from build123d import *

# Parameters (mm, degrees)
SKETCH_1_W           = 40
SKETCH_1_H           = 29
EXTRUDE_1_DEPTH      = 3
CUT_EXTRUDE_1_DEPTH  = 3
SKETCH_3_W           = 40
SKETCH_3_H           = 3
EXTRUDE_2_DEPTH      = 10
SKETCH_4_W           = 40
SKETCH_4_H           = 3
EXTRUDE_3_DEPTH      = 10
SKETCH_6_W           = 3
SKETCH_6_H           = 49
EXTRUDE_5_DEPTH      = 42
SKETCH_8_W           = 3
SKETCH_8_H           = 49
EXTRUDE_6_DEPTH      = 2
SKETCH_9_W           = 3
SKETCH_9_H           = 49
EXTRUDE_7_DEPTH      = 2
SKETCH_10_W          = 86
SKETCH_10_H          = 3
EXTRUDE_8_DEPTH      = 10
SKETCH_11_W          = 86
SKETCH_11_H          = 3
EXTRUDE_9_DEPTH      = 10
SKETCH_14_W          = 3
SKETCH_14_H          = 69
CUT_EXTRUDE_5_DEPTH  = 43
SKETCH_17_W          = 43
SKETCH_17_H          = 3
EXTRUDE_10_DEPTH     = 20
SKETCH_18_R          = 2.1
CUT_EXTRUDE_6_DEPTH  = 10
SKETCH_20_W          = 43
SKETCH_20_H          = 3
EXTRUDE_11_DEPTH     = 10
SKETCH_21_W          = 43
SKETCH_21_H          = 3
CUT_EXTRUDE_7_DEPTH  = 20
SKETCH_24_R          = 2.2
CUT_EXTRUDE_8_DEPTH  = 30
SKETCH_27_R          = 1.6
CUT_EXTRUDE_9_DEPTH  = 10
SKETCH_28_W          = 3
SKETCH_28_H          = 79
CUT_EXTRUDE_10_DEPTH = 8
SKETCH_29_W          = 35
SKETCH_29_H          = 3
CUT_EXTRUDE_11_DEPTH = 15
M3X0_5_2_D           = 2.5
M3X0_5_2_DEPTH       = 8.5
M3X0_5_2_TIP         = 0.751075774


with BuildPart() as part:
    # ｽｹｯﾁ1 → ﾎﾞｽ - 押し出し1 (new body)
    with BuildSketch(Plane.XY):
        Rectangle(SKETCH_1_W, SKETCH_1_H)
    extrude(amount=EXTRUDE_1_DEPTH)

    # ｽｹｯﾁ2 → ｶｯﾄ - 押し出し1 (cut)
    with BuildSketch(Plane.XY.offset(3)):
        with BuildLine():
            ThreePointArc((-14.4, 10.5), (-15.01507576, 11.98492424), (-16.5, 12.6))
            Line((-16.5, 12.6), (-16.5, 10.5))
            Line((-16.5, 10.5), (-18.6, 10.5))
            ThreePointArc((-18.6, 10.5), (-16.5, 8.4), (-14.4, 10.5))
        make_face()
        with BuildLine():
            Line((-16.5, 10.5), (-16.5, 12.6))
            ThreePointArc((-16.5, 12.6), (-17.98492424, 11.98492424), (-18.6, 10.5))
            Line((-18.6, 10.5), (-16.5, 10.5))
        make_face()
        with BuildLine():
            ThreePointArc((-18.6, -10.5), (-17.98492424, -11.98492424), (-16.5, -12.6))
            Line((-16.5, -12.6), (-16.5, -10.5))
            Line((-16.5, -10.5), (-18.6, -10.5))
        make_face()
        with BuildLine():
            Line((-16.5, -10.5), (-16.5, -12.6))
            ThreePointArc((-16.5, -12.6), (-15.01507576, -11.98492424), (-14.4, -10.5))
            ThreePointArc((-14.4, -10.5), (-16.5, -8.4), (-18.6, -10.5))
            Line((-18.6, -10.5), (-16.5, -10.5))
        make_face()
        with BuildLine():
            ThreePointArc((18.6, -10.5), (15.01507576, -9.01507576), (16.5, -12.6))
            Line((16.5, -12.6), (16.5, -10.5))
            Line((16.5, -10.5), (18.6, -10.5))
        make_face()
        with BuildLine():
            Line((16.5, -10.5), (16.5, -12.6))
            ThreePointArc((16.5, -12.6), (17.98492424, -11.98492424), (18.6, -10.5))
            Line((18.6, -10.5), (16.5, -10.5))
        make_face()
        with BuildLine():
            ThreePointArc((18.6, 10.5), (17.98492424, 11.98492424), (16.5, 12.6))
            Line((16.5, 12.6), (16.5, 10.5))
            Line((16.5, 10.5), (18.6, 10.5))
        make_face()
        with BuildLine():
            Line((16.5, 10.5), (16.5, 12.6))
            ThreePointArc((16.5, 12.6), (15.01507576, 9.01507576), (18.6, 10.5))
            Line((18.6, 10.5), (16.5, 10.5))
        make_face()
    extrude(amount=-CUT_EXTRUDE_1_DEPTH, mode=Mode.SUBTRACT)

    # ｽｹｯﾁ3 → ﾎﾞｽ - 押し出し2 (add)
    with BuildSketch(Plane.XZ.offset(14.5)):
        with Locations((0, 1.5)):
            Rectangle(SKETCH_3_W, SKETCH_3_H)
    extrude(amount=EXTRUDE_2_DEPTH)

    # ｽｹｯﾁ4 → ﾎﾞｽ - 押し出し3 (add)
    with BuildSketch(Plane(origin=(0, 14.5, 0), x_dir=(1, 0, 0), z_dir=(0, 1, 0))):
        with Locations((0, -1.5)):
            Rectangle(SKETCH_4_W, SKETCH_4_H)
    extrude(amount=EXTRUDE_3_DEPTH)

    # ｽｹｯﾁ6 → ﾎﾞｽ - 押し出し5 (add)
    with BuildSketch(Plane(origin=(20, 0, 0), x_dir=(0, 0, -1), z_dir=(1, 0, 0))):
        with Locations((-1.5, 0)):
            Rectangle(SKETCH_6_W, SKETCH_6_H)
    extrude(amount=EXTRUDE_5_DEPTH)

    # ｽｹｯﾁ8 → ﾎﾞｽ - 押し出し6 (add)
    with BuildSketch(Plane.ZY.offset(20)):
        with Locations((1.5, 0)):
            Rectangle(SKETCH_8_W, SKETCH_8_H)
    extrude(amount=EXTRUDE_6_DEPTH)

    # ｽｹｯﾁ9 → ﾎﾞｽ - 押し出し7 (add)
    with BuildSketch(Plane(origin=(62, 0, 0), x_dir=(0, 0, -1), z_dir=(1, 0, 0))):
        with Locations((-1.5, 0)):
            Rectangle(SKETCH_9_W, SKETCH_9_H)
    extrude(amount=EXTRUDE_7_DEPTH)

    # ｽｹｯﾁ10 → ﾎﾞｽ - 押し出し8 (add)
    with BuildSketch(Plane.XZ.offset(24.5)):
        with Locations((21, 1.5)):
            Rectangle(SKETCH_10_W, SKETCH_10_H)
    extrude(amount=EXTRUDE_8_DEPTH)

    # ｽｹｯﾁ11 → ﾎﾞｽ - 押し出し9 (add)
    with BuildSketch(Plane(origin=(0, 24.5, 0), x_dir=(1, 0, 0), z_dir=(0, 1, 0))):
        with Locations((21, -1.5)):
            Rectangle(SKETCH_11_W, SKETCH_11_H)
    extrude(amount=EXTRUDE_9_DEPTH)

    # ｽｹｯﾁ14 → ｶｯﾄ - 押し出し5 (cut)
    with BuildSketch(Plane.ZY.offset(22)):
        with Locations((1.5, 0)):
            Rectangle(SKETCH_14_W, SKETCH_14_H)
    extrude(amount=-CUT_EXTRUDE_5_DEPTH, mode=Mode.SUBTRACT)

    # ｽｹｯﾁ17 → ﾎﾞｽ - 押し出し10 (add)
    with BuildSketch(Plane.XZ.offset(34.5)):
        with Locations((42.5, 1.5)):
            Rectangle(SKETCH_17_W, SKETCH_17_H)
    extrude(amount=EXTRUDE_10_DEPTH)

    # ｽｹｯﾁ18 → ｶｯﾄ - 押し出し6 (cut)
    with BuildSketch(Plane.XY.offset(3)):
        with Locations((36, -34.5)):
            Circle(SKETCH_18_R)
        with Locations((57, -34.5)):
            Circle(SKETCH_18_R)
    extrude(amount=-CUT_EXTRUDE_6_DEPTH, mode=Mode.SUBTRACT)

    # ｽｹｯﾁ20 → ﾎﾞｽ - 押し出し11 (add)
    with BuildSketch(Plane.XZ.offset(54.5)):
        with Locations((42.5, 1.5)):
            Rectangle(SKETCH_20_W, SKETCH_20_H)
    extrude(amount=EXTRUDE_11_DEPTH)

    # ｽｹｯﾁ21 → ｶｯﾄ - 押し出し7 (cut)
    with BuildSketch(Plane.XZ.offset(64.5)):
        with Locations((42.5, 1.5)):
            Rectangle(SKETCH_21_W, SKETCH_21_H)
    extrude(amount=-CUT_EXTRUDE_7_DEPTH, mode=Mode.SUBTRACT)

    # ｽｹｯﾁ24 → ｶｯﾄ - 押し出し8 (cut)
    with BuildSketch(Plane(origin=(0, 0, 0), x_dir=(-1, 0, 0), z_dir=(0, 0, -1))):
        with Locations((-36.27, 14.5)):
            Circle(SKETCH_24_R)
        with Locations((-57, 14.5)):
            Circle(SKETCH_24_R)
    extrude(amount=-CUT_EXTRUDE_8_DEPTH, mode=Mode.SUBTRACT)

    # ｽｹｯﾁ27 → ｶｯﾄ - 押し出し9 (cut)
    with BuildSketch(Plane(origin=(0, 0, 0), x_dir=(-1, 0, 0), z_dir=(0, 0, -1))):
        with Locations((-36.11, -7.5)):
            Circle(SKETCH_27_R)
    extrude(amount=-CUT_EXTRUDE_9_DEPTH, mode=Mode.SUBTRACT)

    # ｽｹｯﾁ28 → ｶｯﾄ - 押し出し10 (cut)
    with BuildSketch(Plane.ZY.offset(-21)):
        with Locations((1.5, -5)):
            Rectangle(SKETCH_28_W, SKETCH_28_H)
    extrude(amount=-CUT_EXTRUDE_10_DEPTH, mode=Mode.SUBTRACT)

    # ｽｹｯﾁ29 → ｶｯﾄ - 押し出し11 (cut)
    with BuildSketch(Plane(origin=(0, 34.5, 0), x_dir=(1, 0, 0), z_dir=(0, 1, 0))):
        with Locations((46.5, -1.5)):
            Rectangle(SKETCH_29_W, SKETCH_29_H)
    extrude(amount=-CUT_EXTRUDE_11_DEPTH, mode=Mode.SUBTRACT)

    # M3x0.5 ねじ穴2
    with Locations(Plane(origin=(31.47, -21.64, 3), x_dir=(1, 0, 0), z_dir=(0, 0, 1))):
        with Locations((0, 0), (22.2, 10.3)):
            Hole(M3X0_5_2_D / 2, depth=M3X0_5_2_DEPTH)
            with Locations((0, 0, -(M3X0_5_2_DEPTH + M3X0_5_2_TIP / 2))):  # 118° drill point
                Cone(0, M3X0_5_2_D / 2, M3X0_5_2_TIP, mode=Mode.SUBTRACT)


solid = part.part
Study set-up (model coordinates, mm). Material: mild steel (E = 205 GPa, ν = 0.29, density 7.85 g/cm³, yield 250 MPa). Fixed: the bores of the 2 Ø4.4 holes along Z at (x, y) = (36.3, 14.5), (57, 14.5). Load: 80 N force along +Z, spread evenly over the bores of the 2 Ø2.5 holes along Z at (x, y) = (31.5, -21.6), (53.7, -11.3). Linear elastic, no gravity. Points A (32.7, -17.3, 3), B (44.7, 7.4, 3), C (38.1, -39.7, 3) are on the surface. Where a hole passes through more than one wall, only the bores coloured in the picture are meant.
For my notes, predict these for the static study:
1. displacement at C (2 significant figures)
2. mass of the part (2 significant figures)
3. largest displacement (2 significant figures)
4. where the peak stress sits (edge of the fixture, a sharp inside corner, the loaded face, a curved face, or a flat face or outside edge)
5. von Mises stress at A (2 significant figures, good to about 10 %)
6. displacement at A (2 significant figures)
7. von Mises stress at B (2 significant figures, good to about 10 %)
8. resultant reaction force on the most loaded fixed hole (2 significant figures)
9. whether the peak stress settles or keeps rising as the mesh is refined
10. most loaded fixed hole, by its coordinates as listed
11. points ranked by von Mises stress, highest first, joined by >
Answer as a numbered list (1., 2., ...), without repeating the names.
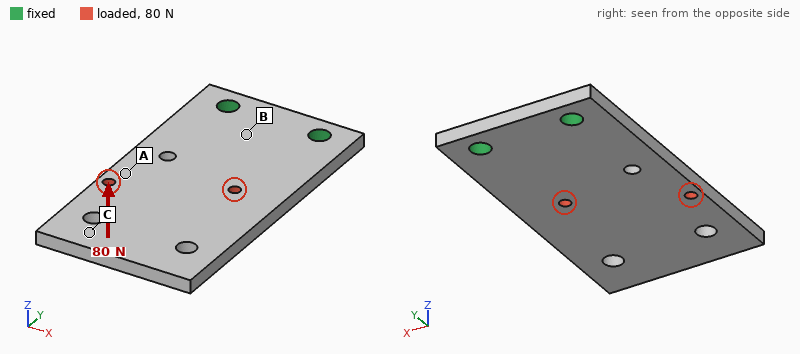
1. 0.10 mm
2. 51 g
3. 0.12 mm
4. edge of the fixture
5. 11 MPa
6. 0.053 mm
7. 31 MPa
8. 53 N
9. keeps rising
10. (36.3, 14.5)
11. B > A > C
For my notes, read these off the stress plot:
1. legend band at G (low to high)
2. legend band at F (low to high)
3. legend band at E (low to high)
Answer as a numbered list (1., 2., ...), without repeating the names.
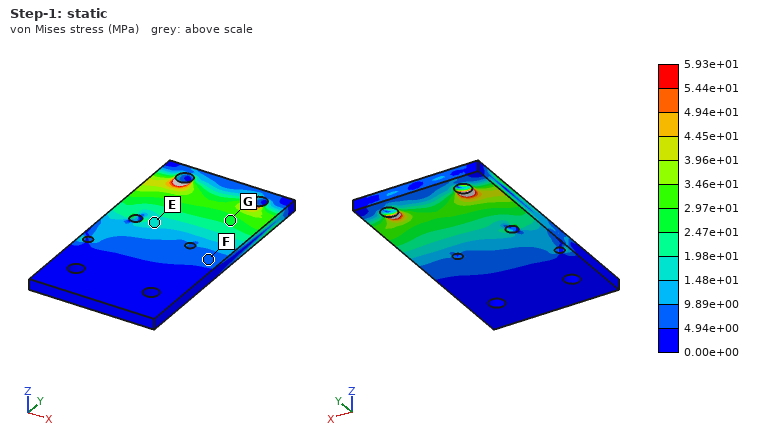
1. 2.47e+01 to 2.97e+01 MPa
2. 4.94e+00 to 9.89e+00 MPa
3. 1.48e+01 to 1.98e+01 MPa
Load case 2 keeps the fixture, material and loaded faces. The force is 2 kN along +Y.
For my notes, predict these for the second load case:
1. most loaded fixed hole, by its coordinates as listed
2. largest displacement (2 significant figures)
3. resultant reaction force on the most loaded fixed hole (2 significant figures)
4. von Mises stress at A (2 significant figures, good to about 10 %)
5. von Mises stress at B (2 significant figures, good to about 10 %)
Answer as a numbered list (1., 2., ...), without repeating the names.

1. (36.3, 14.5)
2. 10 µm
3. 1.4 kN
4. 35 MPa
5. 14 MPa
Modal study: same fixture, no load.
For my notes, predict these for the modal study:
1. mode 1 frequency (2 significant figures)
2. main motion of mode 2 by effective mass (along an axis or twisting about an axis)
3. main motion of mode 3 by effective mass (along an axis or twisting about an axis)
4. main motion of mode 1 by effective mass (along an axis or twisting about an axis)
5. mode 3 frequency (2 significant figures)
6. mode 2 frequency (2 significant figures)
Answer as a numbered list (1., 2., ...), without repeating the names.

1. 740 Hz
2. twisting about Y
3. along Z
4. along Z
5. 4500 Hz
6. 2700 Hz
